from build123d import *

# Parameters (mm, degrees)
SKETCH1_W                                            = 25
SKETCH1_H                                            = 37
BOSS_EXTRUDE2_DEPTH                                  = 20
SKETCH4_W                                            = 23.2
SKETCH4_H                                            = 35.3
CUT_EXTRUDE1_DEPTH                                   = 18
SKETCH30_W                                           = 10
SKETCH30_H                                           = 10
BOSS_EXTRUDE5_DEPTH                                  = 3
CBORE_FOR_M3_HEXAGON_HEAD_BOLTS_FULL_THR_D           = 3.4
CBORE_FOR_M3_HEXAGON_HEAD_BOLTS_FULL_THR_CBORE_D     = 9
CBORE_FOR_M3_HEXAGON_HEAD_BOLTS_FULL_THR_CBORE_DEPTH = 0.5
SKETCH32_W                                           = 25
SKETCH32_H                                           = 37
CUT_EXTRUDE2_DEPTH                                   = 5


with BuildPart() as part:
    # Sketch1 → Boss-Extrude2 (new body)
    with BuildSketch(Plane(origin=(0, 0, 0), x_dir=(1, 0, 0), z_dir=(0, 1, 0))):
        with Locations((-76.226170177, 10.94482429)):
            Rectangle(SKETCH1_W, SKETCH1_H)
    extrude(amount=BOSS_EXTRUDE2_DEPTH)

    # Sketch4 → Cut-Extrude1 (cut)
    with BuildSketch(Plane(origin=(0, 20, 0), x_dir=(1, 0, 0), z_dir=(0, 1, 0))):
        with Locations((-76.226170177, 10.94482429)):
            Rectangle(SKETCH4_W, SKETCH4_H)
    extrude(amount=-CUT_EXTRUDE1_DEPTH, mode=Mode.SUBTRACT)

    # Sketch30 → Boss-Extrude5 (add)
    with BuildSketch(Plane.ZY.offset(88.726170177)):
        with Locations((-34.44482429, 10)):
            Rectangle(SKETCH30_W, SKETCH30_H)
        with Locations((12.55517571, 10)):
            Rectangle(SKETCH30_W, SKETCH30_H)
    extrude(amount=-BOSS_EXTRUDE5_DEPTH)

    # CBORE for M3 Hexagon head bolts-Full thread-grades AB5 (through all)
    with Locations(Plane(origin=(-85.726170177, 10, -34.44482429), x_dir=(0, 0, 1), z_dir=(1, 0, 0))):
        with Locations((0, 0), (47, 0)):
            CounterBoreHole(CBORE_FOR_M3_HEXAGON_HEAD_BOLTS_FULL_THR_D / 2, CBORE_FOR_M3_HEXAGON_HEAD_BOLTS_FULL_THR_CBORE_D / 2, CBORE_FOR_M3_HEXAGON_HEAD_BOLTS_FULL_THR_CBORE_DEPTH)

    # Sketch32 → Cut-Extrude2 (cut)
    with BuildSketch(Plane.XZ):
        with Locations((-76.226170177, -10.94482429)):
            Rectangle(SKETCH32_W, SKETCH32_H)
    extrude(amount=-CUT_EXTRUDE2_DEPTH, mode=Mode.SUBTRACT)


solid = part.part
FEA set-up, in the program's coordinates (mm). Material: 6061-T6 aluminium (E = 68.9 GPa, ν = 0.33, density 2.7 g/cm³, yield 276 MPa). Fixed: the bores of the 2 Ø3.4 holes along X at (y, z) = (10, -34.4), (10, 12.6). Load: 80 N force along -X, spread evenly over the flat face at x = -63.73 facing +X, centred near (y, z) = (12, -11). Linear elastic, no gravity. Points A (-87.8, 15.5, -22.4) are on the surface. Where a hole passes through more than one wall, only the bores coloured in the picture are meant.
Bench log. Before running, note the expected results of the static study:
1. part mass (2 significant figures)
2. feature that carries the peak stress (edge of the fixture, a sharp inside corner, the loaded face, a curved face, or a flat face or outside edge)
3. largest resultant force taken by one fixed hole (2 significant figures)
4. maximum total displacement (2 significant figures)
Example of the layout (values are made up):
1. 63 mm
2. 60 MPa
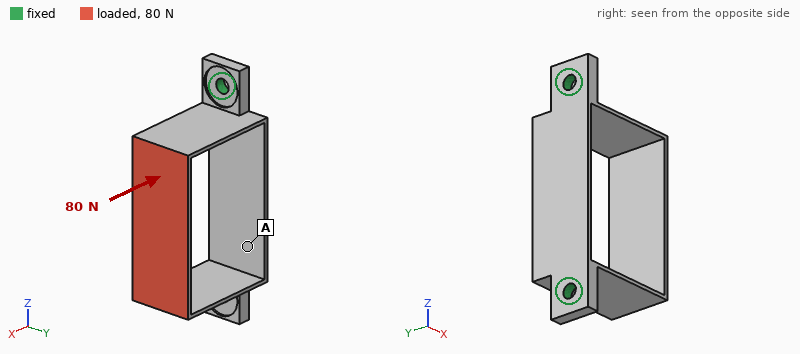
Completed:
1. 5.6 g
2. a flat face or outside edge
3. 42 N
4. 0.31 mm
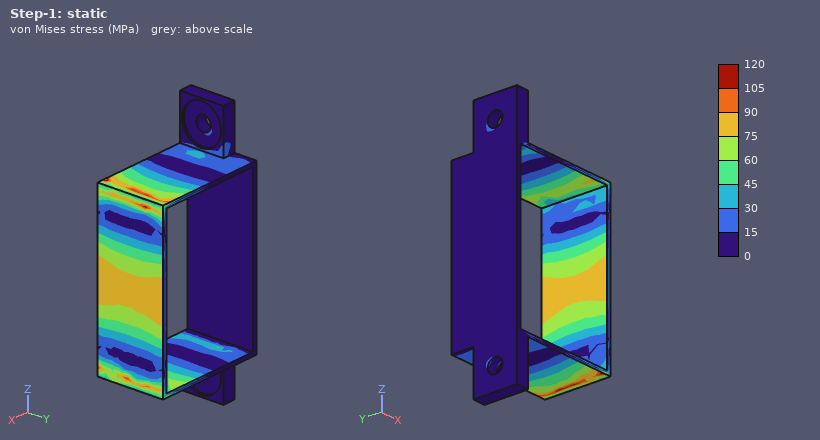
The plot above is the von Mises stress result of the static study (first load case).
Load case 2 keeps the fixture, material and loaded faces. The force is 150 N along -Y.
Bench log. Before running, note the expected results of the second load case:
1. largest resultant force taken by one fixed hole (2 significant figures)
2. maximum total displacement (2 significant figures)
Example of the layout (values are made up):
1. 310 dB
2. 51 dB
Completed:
1. 77 N
2. 0.18 mm
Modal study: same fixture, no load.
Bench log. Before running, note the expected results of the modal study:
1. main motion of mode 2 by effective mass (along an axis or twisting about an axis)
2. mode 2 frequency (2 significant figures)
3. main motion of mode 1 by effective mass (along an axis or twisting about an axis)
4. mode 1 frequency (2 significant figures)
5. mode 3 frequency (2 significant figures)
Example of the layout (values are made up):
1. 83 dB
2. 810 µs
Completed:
1. along X
2. 2500 Hz
3. along Z
4. 1100 Hz
5. 3300 Hz
